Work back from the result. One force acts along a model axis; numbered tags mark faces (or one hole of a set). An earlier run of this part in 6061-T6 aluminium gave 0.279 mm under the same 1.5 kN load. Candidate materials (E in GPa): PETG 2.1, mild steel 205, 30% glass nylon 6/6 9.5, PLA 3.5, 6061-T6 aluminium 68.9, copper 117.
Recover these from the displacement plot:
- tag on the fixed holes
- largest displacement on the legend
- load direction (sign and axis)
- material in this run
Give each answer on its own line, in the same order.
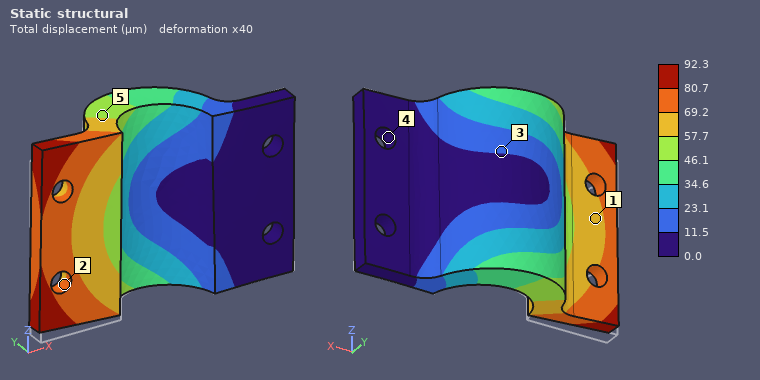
4
92.3 µm
+Z
mild steel
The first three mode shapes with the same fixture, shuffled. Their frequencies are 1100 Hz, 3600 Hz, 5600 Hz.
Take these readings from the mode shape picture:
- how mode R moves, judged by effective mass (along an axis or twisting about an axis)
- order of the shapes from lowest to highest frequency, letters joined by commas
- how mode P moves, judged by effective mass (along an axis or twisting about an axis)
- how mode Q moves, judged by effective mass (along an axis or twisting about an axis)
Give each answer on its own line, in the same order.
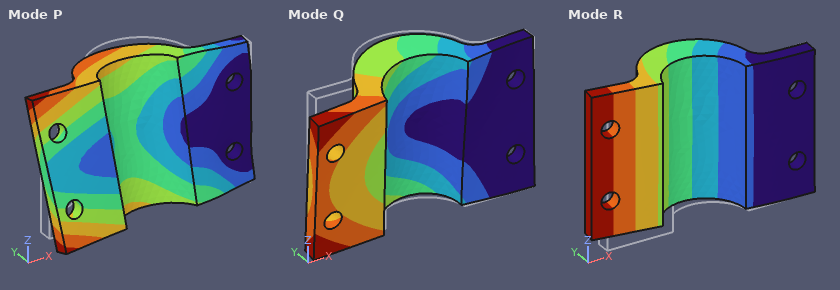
along Y
R, Q, P
along Z
along Z
